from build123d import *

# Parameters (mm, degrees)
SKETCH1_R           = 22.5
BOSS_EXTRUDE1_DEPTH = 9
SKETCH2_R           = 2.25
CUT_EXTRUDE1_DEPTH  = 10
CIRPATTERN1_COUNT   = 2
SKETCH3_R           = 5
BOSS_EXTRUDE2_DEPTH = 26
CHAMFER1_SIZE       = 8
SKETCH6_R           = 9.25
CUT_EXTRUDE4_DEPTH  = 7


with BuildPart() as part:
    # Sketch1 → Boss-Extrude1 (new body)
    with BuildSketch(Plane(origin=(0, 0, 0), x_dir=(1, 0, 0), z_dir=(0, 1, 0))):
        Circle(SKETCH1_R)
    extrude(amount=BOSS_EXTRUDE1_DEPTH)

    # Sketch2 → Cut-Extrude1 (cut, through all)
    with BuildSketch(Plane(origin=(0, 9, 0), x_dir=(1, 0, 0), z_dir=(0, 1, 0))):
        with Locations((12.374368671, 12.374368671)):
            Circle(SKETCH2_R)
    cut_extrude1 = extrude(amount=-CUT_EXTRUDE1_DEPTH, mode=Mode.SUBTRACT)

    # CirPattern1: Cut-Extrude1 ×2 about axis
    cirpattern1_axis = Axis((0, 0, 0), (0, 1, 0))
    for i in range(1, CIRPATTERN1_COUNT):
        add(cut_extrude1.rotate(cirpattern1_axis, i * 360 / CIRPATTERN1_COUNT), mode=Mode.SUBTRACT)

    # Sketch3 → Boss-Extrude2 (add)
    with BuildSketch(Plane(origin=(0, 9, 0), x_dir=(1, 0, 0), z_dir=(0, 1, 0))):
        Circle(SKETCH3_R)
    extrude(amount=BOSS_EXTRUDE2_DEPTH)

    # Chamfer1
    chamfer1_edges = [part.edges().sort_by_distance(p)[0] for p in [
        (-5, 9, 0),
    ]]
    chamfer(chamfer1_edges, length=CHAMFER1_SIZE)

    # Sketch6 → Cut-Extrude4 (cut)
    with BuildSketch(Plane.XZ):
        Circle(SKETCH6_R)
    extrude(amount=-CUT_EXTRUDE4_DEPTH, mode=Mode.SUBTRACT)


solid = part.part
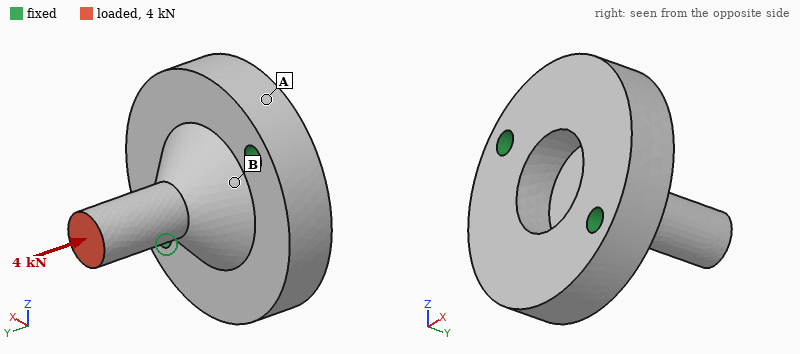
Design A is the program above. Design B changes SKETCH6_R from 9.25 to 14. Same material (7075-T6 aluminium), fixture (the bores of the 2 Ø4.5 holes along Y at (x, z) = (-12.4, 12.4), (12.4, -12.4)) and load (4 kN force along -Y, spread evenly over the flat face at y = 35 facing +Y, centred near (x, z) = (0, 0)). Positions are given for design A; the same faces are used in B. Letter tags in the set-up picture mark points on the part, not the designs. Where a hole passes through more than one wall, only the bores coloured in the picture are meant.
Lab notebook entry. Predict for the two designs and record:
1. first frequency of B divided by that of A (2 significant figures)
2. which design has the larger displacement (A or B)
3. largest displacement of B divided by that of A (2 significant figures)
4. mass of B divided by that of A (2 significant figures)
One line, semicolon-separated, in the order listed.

0.94; B; 1.4; 0.85
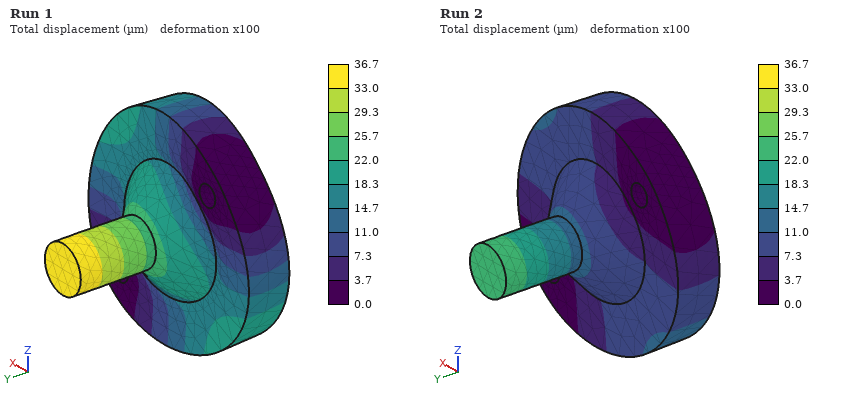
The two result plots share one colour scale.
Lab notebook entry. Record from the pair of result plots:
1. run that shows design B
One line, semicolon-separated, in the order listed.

Run 1
